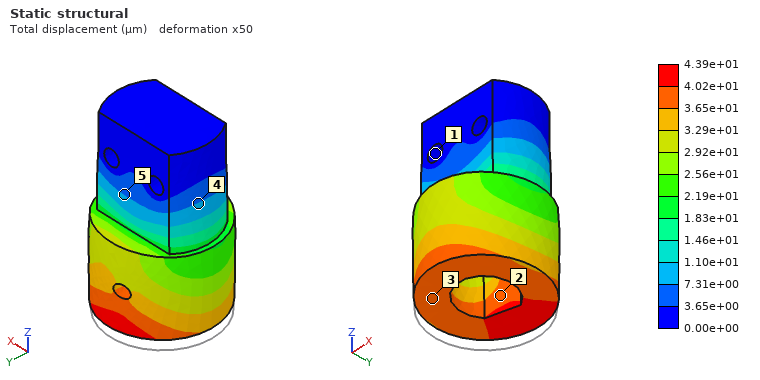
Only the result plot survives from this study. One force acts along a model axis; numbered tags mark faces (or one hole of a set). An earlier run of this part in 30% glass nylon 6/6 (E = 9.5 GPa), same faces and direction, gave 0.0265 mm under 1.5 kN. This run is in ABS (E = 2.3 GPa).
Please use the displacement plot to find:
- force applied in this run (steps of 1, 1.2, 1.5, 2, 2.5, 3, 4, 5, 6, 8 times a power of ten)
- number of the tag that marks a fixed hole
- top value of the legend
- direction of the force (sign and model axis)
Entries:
600 N
1
4.39e+01 µm
+Z
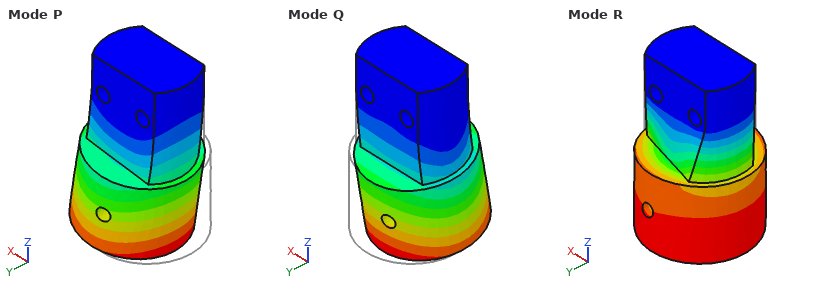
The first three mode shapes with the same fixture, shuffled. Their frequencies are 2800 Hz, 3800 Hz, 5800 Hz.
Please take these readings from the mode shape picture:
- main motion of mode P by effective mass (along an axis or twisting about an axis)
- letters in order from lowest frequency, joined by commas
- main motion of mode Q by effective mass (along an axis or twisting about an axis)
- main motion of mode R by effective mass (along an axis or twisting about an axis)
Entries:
along X
Q, P, R
along Y
twisting about Z
